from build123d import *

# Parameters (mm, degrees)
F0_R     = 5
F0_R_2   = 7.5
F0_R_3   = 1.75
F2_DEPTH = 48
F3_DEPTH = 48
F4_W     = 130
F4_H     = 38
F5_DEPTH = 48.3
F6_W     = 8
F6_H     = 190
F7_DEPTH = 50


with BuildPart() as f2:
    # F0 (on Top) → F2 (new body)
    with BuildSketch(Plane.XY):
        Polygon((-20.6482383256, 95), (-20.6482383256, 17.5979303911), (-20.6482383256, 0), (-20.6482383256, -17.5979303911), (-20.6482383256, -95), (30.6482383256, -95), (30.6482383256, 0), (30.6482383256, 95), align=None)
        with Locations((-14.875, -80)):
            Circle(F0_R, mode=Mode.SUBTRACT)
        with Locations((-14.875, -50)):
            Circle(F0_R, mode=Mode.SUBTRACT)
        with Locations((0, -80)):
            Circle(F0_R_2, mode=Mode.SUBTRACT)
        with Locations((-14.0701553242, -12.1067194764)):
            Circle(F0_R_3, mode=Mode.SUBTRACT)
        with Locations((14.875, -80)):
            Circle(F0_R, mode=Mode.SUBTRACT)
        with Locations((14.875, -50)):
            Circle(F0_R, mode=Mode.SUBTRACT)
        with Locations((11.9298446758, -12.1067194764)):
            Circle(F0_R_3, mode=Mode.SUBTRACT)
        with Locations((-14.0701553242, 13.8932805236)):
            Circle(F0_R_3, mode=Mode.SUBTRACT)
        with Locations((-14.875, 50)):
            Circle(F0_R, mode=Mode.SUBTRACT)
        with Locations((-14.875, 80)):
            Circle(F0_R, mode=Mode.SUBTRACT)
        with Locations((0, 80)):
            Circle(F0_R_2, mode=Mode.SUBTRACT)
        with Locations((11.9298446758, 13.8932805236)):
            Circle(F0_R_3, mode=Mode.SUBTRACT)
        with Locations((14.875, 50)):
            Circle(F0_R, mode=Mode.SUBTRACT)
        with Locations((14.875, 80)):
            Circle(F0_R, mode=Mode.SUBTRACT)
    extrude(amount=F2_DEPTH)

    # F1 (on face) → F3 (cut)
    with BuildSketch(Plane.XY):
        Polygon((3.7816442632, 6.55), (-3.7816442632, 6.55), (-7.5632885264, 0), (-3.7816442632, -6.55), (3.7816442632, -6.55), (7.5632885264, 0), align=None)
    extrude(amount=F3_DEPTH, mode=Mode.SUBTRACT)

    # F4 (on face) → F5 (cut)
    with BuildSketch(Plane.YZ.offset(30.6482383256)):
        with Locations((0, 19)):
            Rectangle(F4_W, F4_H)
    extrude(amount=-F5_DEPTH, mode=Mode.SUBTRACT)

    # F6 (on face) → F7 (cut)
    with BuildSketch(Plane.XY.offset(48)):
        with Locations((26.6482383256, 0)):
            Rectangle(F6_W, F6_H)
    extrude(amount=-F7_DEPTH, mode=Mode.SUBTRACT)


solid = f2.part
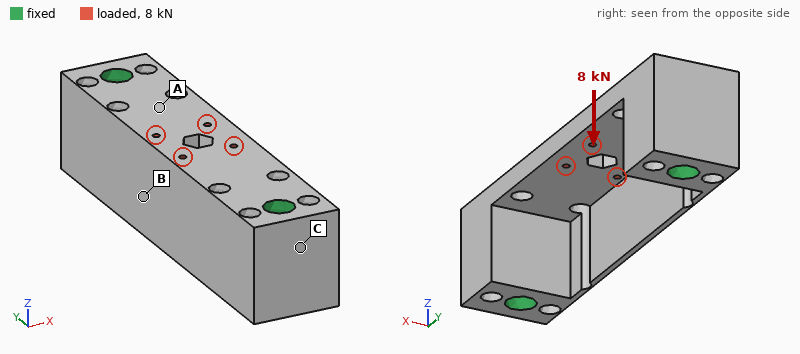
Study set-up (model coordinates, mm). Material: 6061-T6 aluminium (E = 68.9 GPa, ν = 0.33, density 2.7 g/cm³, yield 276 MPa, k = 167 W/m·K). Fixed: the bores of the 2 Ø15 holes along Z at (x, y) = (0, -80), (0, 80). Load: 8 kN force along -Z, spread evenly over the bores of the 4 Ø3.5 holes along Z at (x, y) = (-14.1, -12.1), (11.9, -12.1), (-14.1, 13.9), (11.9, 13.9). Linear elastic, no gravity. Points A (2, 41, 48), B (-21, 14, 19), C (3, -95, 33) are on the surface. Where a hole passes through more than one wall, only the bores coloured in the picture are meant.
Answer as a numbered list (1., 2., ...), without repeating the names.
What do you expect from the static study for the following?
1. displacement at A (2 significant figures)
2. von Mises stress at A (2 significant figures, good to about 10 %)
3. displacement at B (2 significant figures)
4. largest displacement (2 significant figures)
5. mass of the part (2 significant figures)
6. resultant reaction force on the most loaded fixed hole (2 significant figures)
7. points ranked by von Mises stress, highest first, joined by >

1. 0.093 mm
2. 56 MPa
3. 0.12 mm
4. 0.33 mm
5. 430 g
6. 4.1 kN
7. A > B > C
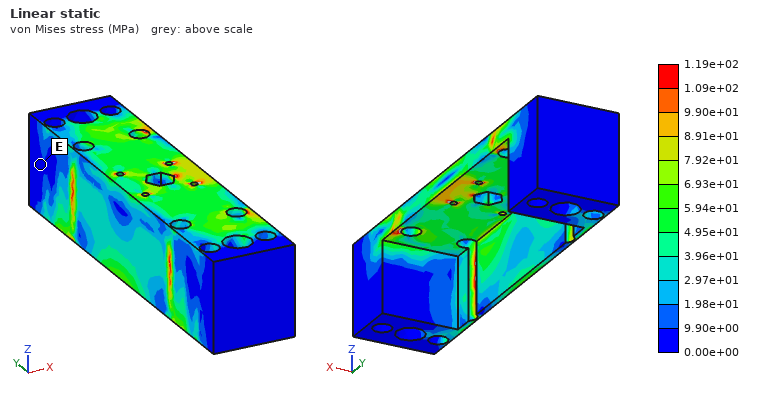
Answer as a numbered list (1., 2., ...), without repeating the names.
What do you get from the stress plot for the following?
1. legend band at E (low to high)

1. 0.00e+00 to 9.90e+00 MPa
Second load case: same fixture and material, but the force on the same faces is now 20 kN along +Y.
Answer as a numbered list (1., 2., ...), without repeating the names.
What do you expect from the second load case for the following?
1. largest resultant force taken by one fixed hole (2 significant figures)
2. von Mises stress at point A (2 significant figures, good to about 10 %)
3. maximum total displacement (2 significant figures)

1. 10 kN
2. 29 MPa
3. 28 µm
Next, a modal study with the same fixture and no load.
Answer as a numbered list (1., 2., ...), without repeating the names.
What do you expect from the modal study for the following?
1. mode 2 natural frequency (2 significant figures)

1. 3400 Hz
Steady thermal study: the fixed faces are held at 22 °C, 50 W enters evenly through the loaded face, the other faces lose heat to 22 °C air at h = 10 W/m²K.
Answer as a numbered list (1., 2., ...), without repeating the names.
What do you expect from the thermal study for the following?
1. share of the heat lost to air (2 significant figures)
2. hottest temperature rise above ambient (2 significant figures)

1. 6.0 %
2. 21 K
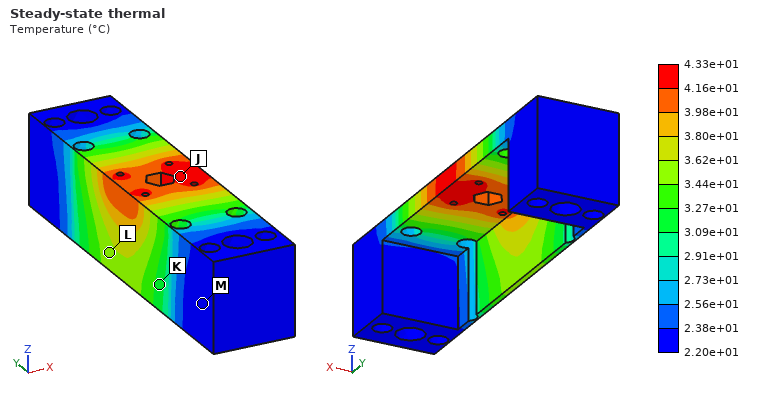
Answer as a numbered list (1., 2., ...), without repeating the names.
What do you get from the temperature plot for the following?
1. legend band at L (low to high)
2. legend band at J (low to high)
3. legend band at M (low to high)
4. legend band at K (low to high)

1. 3.44e+01 to 3.62e+01 °C
2. 4.16e+01 to 4.33e+01 °C
3. 2.20e+01 to 2.38e+01 °C
4. 3.09e+01 to 3.27e+01 °C
